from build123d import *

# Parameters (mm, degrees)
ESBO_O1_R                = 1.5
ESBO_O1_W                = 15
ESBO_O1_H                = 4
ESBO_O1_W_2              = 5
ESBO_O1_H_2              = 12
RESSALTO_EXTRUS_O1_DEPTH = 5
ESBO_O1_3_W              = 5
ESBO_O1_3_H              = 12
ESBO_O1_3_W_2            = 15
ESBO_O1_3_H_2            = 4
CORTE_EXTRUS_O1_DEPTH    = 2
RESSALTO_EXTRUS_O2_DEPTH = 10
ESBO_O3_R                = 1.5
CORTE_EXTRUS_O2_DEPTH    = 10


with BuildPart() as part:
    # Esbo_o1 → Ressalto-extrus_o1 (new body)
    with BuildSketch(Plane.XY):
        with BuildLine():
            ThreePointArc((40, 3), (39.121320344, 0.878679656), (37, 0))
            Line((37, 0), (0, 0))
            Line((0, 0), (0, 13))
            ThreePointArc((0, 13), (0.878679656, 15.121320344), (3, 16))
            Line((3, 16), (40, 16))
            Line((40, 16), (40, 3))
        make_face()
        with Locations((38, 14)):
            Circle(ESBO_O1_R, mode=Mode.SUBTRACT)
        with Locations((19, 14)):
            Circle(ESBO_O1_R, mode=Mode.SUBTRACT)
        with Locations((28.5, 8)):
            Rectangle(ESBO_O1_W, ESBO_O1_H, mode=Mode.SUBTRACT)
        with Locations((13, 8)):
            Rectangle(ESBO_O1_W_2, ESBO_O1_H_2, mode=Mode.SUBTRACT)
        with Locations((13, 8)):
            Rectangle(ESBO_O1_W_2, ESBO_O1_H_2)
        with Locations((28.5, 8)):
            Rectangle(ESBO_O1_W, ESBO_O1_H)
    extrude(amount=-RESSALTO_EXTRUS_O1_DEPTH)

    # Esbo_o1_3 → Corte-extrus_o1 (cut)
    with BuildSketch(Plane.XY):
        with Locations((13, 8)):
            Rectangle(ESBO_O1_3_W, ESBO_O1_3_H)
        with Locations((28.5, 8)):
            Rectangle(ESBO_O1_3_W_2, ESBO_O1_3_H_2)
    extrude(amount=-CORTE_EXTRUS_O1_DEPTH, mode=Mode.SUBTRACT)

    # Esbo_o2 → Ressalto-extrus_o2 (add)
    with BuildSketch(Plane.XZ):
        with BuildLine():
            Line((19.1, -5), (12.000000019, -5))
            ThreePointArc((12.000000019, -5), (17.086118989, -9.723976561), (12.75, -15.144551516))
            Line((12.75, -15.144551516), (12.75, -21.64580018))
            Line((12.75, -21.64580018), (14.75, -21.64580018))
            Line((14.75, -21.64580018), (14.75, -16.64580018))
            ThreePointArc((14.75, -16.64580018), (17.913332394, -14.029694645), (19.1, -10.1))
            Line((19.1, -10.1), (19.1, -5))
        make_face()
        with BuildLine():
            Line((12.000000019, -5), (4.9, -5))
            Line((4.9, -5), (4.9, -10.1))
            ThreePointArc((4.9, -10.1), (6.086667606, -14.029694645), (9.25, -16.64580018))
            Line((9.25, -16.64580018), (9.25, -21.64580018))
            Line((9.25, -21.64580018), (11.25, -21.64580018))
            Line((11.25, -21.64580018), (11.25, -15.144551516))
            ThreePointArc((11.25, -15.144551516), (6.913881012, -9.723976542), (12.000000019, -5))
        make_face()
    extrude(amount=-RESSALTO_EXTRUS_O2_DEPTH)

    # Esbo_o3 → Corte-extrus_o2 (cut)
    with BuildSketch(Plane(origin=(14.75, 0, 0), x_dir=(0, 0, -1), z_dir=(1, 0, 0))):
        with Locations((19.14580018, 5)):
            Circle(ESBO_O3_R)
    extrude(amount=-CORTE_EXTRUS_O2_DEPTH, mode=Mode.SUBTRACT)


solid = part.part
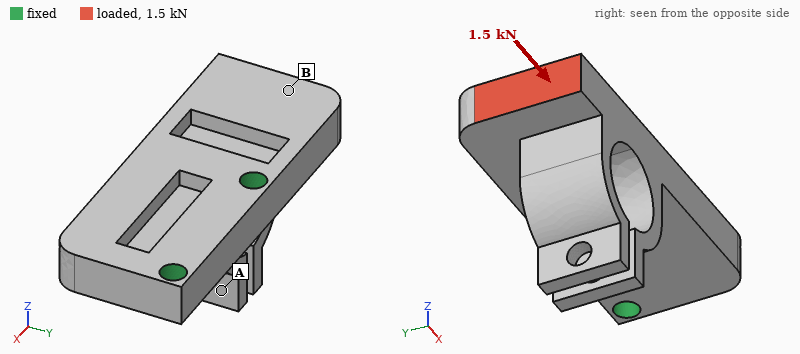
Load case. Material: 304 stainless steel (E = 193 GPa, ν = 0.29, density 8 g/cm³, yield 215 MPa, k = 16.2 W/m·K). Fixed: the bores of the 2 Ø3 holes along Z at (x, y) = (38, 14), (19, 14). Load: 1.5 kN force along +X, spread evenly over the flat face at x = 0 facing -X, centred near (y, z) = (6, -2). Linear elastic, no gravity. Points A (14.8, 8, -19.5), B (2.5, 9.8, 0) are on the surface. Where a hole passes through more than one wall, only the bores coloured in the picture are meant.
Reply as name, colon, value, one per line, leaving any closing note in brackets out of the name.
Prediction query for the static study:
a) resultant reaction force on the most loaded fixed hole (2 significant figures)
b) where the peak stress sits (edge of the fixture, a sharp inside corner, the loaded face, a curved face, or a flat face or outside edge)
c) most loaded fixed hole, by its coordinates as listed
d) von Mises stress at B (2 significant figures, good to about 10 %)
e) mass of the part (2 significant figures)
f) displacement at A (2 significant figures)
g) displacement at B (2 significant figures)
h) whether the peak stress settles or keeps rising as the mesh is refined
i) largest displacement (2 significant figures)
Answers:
resultant reaction force on the most loaded fixed hole: 1.1 kN
where the peak stress sits: edge of the fixture
most loaded fixed hole, by its coordinates as listed: (19, 14)
von Mises stress at B: 21 MPa
mass of the part: 30 g
displacement at A: 2.3 µm
displacement at B: 9.5 µm
whether the peak stress settles or keeps rising as the mesh is refined: keeps rising
largest displacement: 14 µm
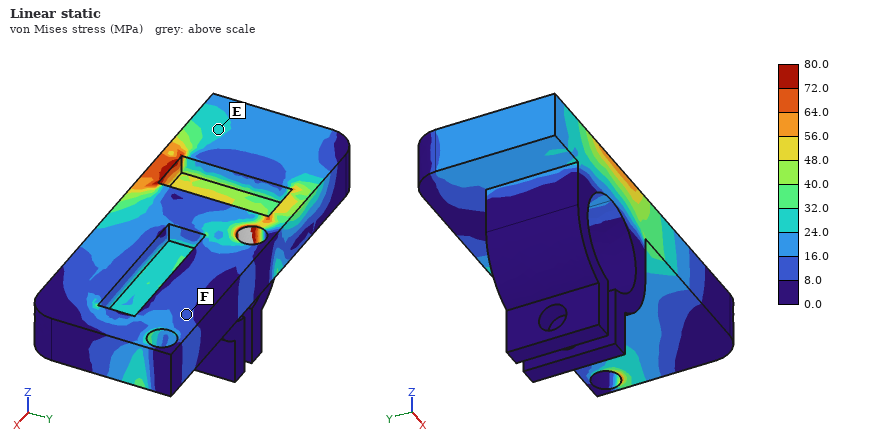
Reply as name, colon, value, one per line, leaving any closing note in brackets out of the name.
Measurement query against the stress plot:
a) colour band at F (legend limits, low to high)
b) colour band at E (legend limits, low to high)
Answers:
colour band at F: 8.0 to 16.0 MPa
colour band at E: 24.0 to 32.0 MPa
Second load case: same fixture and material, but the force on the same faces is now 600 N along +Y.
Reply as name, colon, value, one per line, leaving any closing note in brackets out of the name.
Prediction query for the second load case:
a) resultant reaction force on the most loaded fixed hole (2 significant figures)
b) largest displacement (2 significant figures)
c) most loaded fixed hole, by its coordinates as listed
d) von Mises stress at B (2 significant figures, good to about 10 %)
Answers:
resultant reaction force on the most loaded fixed hole: 1.2 kN
largest displacement: 15 µm
most loaded fixed hole, by its coordinates as listed: (19, 14)
von Mises stress at B: 20 MPa
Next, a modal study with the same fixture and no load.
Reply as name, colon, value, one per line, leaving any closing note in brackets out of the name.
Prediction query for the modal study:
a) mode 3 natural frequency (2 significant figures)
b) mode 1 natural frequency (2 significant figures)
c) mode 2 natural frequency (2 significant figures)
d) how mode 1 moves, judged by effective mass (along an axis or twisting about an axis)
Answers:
mode 3 natural frequency: 7000 Hz
mode 1 natural frequency: 4900 Hz
mode 2 natural frequency: 6300 Hz
how mode 1 moves, judged by effective mass: along Z
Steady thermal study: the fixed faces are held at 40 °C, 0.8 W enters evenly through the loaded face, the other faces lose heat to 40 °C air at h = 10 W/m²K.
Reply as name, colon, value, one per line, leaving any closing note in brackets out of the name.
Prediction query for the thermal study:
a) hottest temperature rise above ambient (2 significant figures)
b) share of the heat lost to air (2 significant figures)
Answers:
hottest temperature rise above ambient: 14 K
share of the heat lost to air: 16 %
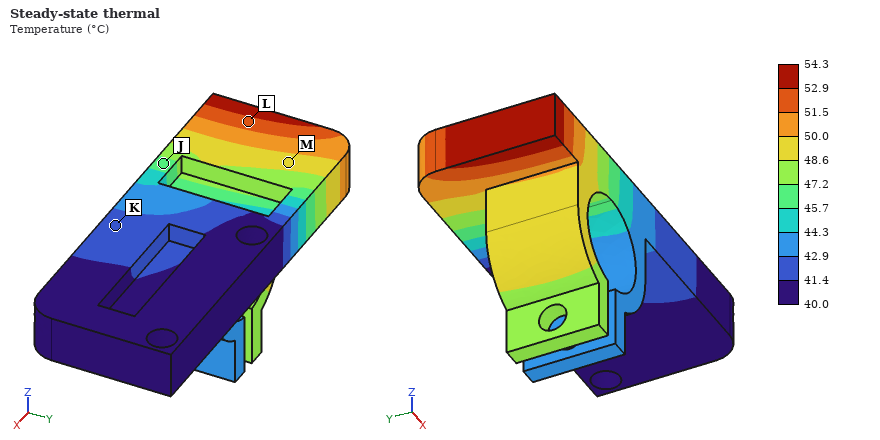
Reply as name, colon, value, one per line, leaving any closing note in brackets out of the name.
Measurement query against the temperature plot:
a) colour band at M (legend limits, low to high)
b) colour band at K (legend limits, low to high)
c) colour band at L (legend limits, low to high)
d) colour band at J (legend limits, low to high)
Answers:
colour band at M: 48.6 to 50.0 °C
colour band at K: 41.4 to 42.9 °C
colour band at L: 51.5 to 52.9 °C
colour band at J: 45.7 to 47.2 °C
